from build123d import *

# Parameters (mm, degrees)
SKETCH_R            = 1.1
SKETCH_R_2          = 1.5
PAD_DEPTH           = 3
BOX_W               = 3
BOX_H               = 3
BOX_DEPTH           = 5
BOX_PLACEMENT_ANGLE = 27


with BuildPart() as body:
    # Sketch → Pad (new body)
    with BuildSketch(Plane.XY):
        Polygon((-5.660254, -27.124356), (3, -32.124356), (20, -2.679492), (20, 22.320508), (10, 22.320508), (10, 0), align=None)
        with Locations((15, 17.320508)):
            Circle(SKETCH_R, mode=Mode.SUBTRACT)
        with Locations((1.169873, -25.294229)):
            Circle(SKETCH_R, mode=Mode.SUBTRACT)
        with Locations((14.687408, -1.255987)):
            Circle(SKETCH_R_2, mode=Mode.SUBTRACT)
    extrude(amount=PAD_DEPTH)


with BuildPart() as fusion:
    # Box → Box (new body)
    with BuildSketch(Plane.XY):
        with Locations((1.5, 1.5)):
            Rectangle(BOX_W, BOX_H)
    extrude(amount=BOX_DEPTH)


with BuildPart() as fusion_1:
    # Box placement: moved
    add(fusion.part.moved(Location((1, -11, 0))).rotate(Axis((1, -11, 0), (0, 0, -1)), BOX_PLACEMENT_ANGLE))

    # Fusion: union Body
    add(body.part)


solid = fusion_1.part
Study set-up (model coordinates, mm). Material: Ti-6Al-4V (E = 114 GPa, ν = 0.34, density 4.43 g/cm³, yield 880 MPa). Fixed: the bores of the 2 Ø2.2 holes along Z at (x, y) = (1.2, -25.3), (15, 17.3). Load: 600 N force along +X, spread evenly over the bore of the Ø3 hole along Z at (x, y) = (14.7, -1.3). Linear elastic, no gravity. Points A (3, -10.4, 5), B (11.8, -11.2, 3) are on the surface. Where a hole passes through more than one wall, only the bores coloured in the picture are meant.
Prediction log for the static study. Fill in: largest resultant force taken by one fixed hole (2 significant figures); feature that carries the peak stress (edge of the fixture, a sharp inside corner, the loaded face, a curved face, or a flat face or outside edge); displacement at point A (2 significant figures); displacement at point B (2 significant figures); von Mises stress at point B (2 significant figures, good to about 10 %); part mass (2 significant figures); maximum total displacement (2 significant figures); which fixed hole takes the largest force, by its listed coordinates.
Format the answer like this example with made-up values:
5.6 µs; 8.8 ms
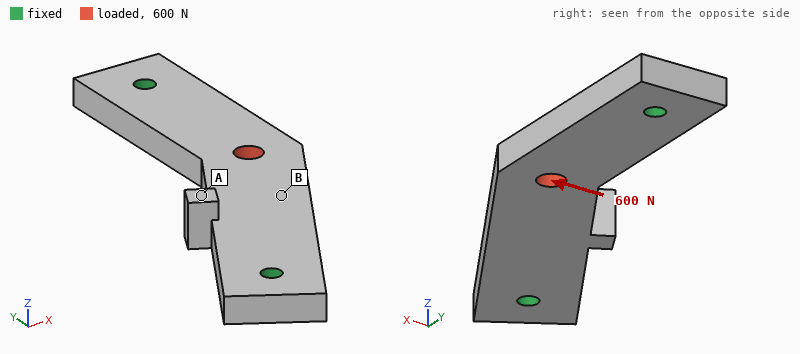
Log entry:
570 N; edge of the fixture; 12 µm; 12 µm; 30 MPa; 7.5 g; 17 µm; (1.2, -25.3)
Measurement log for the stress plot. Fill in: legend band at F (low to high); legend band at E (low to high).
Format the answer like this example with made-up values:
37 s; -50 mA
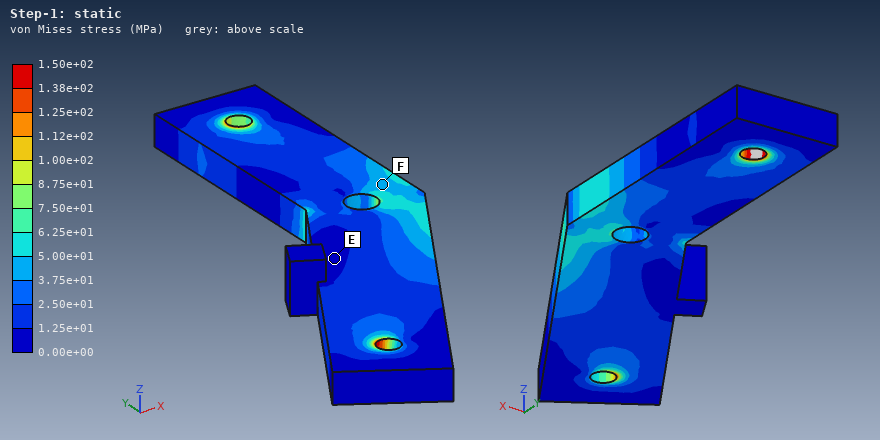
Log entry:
3.75e+01 to 5.00e+01 MPa; 0.00e+00 to 1.25e+01 MPa
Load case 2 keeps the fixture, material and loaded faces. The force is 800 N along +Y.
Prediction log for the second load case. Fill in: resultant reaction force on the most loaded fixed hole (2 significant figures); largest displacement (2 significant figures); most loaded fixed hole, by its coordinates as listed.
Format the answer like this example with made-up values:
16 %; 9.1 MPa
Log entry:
630 N; 6.4 µm; (15, 17.3)
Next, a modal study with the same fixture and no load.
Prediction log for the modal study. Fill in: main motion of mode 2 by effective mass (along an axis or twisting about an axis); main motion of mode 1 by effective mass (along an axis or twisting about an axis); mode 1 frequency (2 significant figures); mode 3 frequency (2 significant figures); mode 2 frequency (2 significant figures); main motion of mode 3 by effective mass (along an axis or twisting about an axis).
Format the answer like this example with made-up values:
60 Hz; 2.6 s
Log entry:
twisting about Y; along Z; 6700 Hz; 17 kHz; 15 kHz; along X
